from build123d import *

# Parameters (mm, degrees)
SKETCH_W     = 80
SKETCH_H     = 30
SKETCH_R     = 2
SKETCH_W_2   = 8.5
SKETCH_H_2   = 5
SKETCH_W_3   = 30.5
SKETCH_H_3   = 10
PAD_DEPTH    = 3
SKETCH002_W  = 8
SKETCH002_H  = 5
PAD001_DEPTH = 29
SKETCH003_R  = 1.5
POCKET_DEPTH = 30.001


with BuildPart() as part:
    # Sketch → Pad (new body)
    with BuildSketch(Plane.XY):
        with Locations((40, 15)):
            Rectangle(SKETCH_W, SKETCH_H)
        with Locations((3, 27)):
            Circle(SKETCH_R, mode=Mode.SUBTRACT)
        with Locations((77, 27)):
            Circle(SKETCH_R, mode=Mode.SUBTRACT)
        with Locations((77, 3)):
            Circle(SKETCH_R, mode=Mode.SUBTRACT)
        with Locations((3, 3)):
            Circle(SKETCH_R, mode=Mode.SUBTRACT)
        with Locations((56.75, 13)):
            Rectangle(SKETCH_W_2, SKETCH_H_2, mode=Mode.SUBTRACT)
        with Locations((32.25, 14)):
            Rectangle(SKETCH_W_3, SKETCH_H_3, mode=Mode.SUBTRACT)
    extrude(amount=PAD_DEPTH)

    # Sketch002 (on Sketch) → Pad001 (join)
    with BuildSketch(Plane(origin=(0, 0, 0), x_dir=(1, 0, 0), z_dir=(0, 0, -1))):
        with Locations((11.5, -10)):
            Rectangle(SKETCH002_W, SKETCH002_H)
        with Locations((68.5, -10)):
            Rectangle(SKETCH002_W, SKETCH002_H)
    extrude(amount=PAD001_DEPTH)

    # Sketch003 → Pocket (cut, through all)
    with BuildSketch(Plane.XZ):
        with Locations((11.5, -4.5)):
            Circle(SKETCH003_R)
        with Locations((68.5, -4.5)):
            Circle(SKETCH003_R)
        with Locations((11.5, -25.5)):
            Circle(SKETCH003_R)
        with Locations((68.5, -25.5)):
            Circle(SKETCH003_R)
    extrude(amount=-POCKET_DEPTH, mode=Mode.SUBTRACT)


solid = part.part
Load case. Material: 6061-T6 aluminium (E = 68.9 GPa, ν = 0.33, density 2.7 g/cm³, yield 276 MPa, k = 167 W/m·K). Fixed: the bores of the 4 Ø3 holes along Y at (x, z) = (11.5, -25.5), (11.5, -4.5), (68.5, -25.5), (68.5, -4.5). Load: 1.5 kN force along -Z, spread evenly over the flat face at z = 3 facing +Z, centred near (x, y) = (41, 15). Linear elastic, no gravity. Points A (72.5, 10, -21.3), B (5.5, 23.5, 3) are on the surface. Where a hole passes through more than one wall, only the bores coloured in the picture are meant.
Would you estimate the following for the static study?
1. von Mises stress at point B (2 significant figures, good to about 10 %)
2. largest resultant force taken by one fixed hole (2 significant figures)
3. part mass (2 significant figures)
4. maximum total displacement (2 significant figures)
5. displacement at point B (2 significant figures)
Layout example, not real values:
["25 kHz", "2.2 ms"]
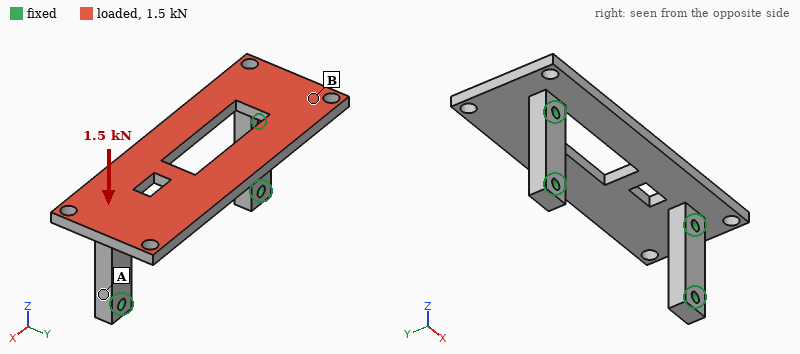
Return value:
["48 MPa", "810 N", "22 g", "0.39 mm", "0.11 mm"]
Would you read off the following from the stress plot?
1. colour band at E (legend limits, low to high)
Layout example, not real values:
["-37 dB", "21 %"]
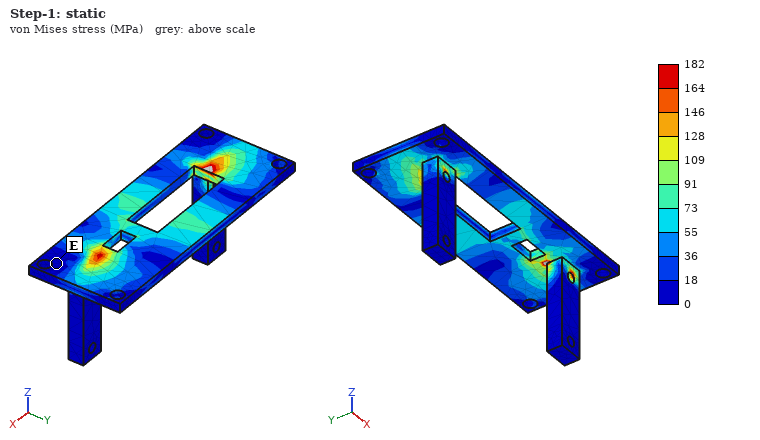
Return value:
["0 to 18 MPa"]
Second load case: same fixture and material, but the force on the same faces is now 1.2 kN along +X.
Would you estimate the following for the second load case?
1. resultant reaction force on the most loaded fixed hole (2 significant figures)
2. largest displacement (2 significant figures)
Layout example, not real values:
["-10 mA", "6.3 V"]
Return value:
["700 N", "27 µm"]
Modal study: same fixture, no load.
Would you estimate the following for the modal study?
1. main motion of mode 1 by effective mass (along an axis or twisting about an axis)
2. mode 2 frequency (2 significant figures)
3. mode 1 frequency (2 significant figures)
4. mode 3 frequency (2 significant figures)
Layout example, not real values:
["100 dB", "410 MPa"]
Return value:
["along Z", "5000 Hz", "3100 Hz", "5500 Hz"]
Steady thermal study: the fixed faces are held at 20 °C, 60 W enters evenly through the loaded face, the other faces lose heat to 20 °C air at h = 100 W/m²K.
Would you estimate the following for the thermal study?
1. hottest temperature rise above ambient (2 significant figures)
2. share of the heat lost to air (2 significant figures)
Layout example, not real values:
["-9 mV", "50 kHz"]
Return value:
["47 K", "17 %"]
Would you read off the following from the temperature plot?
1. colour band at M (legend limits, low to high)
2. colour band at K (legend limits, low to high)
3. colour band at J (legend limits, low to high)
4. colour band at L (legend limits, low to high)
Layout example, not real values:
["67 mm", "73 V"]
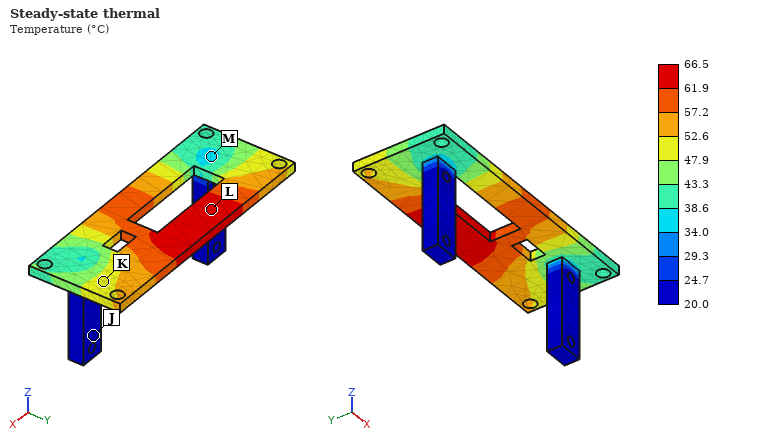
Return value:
["34.0 to 38.6 °C", "47.9 to 52.6 °C", "20.0 to 24.7 °C", "61.9 to 66.5 °C"]
